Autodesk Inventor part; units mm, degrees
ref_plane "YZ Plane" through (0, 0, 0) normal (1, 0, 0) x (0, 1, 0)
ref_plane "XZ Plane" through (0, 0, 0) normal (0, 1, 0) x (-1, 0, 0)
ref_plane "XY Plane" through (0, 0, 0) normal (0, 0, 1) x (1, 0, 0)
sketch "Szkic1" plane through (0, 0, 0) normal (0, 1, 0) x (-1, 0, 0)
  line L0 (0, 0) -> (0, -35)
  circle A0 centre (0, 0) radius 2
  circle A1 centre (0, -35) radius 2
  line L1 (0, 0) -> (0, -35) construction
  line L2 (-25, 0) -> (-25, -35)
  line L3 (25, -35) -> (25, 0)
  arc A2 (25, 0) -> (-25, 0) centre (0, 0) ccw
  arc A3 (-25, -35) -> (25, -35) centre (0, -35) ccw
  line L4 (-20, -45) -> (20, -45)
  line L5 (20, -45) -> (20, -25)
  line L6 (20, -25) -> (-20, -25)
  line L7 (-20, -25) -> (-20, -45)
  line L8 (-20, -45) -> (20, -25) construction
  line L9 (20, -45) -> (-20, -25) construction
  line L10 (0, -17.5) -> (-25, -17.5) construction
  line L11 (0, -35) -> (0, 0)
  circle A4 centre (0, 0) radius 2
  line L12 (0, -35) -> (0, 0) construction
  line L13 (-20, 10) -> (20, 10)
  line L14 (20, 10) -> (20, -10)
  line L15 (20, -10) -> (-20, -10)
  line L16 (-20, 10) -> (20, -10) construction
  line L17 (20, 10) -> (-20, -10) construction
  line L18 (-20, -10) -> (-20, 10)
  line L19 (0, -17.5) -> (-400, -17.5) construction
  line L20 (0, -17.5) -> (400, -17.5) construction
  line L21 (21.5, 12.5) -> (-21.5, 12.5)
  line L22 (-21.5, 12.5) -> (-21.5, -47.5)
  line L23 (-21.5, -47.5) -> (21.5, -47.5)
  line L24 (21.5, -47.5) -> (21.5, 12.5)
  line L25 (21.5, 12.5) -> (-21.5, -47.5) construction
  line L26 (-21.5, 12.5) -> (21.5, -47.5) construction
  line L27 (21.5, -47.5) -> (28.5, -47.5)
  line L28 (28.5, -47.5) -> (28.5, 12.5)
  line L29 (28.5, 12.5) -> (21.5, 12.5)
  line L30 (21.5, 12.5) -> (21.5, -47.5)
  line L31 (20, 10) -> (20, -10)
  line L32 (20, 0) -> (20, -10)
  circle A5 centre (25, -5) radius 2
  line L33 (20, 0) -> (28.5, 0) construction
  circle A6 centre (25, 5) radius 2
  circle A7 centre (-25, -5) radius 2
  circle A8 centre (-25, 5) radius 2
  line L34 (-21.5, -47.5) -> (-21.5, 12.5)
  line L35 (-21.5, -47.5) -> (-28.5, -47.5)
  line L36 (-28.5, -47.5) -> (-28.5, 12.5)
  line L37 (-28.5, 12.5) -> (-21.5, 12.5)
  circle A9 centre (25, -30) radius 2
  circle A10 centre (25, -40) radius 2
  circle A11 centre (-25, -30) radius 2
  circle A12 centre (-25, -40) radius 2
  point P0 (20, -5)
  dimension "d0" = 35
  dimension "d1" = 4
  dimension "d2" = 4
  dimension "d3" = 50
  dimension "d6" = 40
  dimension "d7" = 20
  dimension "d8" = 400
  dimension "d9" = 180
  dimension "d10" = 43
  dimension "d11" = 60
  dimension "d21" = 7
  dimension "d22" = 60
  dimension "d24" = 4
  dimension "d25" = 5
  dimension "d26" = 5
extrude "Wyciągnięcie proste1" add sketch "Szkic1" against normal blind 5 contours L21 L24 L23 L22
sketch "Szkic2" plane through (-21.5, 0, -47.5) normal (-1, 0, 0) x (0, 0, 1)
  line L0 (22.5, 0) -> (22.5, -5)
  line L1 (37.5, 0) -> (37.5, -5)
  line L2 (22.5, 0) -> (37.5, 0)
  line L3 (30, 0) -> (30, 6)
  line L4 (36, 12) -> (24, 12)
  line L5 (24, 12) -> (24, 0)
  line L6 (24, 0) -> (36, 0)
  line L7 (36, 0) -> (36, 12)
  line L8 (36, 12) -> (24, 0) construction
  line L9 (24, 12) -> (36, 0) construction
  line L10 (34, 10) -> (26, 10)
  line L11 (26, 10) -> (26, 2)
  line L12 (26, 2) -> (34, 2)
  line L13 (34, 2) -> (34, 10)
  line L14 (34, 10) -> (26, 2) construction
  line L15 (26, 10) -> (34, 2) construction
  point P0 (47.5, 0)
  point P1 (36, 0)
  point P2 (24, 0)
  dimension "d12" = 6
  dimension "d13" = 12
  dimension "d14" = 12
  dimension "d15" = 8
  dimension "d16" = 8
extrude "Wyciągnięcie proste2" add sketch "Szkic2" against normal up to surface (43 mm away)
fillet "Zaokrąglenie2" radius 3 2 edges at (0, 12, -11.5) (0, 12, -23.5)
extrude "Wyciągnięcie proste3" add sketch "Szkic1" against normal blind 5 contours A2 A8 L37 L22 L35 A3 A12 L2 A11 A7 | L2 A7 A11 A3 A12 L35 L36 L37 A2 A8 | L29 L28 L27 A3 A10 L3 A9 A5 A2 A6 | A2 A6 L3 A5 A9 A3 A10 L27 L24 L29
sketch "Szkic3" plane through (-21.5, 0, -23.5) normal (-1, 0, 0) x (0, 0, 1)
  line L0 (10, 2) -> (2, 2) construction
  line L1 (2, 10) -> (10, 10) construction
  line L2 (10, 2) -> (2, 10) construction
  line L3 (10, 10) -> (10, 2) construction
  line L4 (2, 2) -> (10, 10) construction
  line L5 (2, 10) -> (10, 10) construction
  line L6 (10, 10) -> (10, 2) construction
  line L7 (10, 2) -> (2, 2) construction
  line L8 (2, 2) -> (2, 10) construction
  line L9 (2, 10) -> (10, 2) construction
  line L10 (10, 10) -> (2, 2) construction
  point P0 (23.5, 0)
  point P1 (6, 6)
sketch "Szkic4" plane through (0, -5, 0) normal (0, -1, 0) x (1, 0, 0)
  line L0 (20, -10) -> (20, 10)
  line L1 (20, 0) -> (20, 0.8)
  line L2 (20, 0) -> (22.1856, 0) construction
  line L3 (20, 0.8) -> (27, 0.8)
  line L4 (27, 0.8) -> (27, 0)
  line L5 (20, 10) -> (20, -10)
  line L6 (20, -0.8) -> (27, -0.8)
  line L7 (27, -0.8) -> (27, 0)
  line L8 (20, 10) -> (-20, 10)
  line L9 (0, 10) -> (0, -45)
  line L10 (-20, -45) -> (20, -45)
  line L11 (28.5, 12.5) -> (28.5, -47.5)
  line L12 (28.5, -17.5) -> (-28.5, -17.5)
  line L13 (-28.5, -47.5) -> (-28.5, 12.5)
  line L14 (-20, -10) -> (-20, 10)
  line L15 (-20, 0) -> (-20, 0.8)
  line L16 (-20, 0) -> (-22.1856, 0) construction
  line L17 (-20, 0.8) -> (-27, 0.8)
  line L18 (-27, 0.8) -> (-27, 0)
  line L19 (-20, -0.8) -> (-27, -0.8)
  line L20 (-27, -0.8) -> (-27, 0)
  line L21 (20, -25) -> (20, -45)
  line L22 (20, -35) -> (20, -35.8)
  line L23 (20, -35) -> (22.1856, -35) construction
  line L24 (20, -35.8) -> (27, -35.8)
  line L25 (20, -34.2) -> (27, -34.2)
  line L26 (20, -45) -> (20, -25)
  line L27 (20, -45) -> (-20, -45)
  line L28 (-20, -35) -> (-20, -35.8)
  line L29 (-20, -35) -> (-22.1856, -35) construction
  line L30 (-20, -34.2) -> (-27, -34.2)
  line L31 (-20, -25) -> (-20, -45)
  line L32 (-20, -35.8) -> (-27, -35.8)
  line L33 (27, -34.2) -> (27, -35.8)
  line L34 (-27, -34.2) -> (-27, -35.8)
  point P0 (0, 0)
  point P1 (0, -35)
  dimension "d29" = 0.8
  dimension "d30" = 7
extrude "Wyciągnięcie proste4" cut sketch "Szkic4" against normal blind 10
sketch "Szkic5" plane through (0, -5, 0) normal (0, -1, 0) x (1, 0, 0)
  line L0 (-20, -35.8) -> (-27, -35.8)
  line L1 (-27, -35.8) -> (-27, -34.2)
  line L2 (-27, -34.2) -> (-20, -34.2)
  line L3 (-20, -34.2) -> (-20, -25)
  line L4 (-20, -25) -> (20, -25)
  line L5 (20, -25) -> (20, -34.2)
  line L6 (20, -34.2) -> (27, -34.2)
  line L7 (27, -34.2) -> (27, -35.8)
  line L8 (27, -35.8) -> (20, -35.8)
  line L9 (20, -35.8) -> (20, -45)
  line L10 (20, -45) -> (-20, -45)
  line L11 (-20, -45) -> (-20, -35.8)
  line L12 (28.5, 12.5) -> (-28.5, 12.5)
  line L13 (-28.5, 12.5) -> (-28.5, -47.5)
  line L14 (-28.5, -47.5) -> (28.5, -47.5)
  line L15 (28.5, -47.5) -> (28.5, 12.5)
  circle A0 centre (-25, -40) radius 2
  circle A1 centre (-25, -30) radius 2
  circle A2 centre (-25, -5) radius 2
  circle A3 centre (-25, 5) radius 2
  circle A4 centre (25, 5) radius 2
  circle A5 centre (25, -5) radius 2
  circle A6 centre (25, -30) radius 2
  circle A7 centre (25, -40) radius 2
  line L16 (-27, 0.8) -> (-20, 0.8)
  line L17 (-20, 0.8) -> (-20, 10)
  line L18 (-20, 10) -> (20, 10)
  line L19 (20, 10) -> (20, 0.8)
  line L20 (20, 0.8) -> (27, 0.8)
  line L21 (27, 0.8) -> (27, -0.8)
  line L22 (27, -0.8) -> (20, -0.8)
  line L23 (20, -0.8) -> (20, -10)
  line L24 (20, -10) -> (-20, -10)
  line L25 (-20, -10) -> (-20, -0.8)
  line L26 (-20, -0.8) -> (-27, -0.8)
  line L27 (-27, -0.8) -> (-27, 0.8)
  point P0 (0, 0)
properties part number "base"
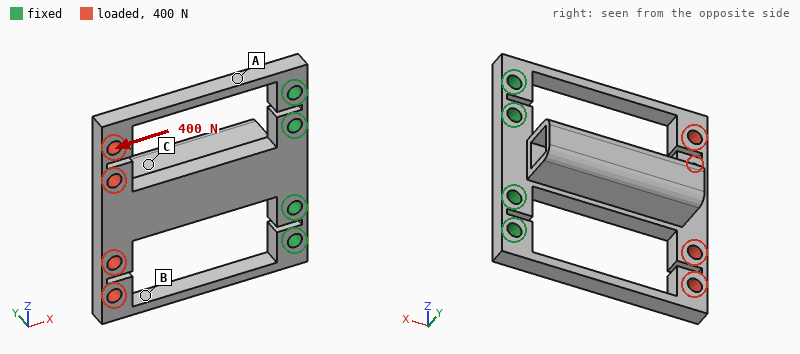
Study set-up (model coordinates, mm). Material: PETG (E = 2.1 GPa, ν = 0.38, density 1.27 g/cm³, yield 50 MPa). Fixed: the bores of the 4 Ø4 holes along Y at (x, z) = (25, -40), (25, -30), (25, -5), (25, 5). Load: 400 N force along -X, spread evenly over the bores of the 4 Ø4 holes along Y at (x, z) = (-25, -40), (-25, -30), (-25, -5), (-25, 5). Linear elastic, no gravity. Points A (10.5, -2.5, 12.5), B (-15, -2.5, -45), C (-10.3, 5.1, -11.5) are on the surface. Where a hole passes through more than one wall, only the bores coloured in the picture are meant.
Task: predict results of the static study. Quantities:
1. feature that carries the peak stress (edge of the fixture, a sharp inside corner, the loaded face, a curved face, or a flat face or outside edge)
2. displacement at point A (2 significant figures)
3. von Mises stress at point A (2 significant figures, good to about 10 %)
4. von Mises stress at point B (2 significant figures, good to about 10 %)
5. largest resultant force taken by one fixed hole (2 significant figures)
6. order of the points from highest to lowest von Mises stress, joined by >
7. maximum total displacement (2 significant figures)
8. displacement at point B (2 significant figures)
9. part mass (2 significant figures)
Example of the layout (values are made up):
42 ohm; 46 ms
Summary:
a flat face or outside edge; 0.15 mm; 5.2 MPa; 11 MPa; 160 N; B > A > C; 0.50 mm; 0.39 mm; 15 g
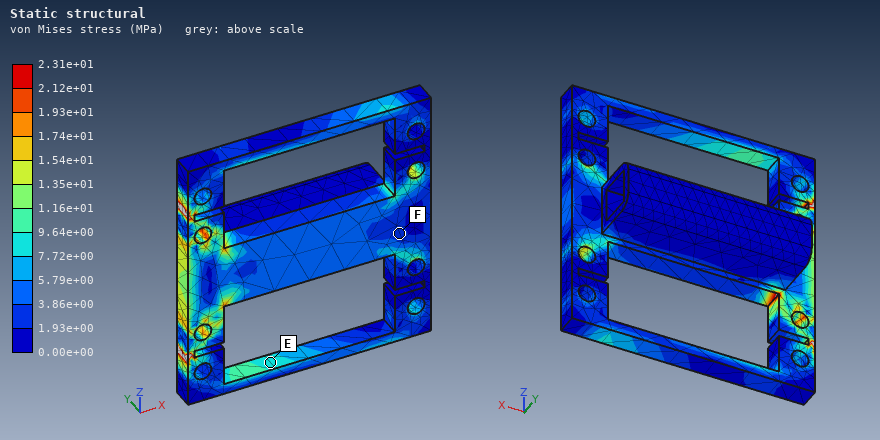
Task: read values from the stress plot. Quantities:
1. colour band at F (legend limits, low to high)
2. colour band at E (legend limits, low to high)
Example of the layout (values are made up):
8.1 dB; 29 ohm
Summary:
1.93e+00 to 3.86e+00 MPa; 7.72e+00 to 9.64e+00 MPa
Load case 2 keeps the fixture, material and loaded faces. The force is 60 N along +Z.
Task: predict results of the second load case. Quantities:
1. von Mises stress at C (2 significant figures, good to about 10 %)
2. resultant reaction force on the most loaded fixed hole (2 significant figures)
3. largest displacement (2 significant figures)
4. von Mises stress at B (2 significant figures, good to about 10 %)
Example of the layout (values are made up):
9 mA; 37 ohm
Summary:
1.7 MPa; 120 N; 0.84 mm; 9.1 MPa
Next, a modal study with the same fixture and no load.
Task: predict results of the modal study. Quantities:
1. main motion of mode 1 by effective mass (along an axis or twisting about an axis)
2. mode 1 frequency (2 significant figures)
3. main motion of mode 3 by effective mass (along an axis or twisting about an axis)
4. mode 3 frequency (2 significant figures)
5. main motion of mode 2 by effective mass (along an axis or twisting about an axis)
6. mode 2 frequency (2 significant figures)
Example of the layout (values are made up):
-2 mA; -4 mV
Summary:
along Y; 290 Hz; twisting about X; 760 Hz; along Z; 660 Hz
